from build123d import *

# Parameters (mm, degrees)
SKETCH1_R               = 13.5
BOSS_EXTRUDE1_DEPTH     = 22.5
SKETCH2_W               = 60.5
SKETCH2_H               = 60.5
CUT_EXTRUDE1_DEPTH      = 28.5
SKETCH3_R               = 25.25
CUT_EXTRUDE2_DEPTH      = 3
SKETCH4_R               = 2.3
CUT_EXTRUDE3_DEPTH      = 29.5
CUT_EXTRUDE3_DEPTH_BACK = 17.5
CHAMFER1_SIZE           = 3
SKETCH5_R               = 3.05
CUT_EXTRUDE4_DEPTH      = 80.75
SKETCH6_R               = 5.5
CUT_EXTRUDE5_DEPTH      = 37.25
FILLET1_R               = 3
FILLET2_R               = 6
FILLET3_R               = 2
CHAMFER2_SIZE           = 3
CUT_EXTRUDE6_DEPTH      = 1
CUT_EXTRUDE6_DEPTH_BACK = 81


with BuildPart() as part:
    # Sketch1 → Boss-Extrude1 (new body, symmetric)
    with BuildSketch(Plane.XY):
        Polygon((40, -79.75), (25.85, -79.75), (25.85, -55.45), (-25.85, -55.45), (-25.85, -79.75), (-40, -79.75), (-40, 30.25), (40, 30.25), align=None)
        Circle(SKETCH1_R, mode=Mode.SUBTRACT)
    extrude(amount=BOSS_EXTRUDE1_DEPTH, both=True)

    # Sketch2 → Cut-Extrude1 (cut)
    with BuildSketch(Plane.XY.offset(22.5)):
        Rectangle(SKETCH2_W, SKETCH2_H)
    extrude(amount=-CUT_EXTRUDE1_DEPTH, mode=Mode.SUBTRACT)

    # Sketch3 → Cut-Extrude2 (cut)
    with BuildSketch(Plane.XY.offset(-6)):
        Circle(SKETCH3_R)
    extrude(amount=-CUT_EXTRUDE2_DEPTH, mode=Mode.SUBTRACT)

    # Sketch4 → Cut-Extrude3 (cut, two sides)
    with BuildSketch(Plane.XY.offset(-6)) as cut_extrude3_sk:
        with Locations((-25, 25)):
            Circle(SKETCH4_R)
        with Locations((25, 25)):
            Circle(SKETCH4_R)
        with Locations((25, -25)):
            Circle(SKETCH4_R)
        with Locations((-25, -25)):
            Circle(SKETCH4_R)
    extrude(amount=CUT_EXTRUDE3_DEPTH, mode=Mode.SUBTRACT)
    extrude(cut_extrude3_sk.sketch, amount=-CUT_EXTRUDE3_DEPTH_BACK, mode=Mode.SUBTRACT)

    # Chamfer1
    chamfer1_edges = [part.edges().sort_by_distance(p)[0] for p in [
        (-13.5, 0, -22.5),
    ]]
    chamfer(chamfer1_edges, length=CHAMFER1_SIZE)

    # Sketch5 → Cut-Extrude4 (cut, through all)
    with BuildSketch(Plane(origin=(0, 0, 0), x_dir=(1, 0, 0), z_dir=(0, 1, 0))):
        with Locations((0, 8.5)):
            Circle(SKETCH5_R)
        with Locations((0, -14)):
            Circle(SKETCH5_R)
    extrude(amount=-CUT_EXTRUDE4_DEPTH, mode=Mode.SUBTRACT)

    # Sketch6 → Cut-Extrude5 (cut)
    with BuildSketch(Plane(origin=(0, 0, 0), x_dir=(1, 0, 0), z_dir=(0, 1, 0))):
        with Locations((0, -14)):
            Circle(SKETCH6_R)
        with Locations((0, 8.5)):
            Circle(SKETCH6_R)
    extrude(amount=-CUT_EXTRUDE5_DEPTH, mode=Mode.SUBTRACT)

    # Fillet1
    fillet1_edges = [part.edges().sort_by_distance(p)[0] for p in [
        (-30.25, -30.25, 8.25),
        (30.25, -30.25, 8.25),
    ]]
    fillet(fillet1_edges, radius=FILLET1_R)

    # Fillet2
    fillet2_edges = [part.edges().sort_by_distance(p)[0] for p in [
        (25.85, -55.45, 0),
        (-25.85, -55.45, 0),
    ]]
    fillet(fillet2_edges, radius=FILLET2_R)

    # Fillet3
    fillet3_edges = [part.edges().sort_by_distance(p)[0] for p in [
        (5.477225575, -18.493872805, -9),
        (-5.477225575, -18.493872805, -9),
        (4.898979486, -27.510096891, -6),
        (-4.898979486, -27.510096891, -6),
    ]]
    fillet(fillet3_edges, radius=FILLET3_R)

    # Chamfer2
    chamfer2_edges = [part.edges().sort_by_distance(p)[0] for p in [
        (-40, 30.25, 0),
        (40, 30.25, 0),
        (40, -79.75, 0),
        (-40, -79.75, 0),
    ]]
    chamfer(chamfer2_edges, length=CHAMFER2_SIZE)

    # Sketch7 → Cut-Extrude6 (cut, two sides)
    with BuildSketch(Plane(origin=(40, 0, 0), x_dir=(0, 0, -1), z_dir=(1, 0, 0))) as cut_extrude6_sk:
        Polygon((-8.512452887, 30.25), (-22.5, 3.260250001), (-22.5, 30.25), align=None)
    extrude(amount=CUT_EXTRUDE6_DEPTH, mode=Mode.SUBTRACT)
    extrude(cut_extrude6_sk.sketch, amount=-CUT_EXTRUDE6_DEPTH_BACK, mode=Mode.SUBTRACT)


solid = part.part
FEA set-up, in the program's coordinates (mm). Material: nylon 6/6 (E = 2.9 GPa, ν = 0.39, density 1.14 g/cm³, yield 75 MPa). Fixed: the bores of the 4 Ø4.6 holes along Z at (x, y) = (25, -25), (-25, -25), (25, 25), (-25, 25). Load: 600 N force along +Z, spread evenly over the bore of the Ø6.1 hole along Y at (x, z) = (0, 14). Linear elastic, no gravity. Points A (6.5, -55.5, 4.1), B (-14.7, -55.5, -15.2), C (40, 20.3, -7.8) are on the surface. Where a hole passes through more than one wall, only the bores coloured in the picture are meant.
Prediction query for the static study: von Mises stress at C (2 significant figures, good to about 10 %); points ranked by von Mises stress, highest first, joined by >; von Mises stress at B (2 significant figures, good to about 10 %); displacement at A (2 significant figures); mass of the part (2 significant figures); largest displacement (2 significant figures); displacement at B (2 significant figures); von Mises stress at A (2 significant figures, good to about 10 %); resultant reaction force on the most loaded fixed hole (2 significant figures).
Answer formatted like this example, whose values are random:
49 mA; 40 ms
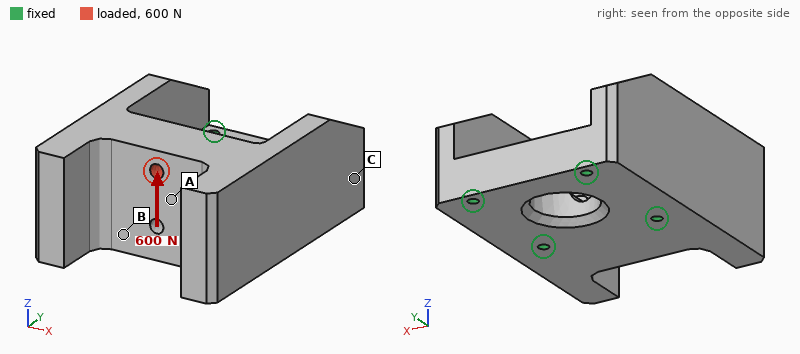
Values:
0.36 MPa; A > B > C; 0.69 MPa; 46 µm; 240 g; 63 µm; 37 µm; 1.3 MPa; 390 N
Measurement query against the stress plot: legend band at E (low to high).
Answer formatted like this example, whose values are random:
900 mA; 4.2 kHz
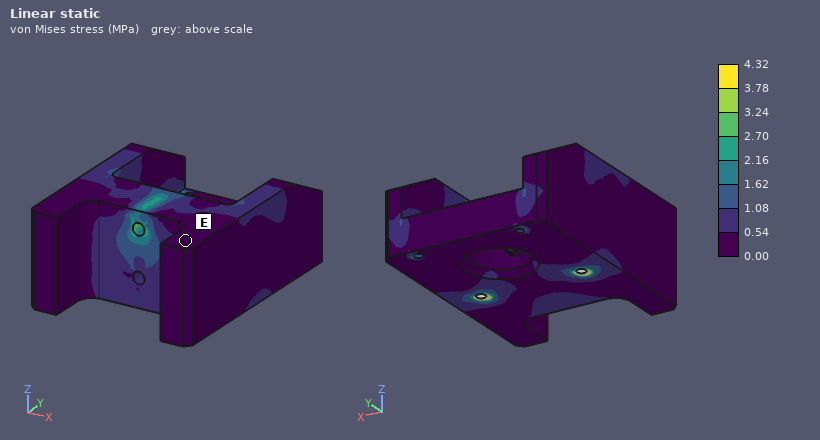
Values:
0.00 to 0.54 MPa
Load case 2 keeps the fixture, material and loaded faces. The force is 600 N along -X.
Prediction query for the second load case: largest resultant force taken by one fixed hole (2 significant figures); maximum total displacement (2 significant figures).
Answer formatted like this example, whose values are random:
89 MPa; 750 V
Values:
450 N; 44 µm
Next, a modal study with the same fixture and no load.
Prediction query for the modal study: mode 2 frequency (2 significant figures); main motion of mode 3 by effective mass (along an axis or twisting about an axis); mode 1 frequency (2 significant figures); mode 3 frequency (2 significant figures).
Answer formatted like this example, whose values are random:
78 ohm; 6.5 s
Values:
1800 Hz; along X; 1500 Hz; 2300 Hz
